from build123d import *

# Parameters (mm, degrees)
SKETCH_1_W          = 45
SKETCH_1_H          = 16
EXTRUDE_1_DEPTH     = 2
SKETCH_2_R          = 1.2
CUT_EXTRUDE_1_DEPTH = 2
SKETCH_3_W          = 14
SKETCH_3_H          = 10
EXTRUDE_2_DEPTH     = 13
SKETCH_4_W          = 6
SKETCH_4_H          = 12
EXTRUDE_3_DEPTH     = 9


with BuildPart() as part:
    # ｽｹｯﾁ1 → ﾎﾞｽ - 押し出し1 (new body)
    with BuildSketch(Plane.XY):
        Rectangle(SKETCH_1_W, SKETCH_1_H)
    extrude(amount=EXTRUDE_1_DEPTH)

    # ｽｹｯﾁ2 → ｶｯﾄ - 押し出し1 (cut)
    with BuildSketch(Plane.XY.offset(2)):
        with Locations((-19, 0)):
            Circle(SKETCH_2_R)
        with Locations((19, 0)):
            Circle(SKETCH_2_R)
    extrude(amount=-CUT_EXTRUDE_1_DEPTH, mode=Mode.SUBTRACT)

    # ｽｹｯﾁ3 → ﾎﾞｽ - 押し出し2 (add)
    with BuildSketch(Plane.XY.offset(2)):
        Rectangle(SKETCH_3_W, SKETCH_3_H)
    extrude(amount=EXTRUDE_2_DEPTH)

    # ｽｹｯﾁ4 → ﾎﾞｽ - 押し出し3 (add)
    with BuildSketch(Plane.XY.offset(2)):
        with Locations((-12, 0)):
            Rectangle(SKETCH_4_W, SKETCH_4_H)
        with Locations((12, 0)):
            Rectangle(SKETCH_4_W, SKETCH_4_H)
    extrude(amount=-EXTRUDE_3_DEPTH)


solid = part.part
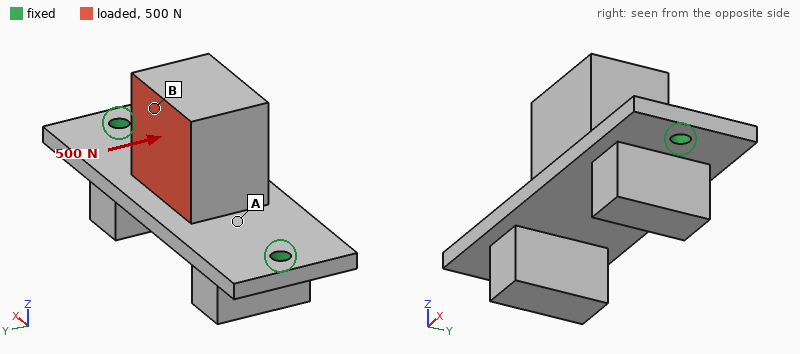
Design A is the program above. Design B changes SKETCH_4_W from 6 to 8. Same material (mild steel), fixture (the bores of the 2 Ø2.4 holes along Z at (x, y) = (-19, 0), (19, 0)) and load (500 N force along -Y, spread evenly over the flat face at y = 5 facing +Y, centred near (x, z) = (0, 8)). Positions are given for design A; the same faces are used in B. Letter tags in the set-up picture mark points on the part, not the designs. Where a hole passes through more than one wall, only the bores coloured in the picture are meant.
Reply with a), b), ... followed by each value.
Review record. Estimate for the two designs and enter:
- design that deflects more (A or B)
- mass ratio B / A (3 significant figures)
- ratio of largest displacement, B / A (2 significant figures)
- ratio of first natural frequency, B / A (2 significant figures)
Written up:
a) A
b) 1.08
c) 0.81
d) 1.1
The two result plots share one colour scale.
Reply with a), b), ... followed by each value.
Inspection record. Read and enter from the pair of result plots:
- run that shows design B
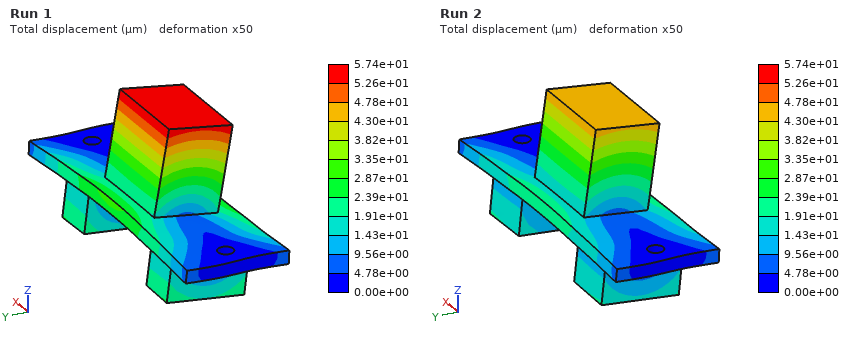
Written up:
a) Run 2
